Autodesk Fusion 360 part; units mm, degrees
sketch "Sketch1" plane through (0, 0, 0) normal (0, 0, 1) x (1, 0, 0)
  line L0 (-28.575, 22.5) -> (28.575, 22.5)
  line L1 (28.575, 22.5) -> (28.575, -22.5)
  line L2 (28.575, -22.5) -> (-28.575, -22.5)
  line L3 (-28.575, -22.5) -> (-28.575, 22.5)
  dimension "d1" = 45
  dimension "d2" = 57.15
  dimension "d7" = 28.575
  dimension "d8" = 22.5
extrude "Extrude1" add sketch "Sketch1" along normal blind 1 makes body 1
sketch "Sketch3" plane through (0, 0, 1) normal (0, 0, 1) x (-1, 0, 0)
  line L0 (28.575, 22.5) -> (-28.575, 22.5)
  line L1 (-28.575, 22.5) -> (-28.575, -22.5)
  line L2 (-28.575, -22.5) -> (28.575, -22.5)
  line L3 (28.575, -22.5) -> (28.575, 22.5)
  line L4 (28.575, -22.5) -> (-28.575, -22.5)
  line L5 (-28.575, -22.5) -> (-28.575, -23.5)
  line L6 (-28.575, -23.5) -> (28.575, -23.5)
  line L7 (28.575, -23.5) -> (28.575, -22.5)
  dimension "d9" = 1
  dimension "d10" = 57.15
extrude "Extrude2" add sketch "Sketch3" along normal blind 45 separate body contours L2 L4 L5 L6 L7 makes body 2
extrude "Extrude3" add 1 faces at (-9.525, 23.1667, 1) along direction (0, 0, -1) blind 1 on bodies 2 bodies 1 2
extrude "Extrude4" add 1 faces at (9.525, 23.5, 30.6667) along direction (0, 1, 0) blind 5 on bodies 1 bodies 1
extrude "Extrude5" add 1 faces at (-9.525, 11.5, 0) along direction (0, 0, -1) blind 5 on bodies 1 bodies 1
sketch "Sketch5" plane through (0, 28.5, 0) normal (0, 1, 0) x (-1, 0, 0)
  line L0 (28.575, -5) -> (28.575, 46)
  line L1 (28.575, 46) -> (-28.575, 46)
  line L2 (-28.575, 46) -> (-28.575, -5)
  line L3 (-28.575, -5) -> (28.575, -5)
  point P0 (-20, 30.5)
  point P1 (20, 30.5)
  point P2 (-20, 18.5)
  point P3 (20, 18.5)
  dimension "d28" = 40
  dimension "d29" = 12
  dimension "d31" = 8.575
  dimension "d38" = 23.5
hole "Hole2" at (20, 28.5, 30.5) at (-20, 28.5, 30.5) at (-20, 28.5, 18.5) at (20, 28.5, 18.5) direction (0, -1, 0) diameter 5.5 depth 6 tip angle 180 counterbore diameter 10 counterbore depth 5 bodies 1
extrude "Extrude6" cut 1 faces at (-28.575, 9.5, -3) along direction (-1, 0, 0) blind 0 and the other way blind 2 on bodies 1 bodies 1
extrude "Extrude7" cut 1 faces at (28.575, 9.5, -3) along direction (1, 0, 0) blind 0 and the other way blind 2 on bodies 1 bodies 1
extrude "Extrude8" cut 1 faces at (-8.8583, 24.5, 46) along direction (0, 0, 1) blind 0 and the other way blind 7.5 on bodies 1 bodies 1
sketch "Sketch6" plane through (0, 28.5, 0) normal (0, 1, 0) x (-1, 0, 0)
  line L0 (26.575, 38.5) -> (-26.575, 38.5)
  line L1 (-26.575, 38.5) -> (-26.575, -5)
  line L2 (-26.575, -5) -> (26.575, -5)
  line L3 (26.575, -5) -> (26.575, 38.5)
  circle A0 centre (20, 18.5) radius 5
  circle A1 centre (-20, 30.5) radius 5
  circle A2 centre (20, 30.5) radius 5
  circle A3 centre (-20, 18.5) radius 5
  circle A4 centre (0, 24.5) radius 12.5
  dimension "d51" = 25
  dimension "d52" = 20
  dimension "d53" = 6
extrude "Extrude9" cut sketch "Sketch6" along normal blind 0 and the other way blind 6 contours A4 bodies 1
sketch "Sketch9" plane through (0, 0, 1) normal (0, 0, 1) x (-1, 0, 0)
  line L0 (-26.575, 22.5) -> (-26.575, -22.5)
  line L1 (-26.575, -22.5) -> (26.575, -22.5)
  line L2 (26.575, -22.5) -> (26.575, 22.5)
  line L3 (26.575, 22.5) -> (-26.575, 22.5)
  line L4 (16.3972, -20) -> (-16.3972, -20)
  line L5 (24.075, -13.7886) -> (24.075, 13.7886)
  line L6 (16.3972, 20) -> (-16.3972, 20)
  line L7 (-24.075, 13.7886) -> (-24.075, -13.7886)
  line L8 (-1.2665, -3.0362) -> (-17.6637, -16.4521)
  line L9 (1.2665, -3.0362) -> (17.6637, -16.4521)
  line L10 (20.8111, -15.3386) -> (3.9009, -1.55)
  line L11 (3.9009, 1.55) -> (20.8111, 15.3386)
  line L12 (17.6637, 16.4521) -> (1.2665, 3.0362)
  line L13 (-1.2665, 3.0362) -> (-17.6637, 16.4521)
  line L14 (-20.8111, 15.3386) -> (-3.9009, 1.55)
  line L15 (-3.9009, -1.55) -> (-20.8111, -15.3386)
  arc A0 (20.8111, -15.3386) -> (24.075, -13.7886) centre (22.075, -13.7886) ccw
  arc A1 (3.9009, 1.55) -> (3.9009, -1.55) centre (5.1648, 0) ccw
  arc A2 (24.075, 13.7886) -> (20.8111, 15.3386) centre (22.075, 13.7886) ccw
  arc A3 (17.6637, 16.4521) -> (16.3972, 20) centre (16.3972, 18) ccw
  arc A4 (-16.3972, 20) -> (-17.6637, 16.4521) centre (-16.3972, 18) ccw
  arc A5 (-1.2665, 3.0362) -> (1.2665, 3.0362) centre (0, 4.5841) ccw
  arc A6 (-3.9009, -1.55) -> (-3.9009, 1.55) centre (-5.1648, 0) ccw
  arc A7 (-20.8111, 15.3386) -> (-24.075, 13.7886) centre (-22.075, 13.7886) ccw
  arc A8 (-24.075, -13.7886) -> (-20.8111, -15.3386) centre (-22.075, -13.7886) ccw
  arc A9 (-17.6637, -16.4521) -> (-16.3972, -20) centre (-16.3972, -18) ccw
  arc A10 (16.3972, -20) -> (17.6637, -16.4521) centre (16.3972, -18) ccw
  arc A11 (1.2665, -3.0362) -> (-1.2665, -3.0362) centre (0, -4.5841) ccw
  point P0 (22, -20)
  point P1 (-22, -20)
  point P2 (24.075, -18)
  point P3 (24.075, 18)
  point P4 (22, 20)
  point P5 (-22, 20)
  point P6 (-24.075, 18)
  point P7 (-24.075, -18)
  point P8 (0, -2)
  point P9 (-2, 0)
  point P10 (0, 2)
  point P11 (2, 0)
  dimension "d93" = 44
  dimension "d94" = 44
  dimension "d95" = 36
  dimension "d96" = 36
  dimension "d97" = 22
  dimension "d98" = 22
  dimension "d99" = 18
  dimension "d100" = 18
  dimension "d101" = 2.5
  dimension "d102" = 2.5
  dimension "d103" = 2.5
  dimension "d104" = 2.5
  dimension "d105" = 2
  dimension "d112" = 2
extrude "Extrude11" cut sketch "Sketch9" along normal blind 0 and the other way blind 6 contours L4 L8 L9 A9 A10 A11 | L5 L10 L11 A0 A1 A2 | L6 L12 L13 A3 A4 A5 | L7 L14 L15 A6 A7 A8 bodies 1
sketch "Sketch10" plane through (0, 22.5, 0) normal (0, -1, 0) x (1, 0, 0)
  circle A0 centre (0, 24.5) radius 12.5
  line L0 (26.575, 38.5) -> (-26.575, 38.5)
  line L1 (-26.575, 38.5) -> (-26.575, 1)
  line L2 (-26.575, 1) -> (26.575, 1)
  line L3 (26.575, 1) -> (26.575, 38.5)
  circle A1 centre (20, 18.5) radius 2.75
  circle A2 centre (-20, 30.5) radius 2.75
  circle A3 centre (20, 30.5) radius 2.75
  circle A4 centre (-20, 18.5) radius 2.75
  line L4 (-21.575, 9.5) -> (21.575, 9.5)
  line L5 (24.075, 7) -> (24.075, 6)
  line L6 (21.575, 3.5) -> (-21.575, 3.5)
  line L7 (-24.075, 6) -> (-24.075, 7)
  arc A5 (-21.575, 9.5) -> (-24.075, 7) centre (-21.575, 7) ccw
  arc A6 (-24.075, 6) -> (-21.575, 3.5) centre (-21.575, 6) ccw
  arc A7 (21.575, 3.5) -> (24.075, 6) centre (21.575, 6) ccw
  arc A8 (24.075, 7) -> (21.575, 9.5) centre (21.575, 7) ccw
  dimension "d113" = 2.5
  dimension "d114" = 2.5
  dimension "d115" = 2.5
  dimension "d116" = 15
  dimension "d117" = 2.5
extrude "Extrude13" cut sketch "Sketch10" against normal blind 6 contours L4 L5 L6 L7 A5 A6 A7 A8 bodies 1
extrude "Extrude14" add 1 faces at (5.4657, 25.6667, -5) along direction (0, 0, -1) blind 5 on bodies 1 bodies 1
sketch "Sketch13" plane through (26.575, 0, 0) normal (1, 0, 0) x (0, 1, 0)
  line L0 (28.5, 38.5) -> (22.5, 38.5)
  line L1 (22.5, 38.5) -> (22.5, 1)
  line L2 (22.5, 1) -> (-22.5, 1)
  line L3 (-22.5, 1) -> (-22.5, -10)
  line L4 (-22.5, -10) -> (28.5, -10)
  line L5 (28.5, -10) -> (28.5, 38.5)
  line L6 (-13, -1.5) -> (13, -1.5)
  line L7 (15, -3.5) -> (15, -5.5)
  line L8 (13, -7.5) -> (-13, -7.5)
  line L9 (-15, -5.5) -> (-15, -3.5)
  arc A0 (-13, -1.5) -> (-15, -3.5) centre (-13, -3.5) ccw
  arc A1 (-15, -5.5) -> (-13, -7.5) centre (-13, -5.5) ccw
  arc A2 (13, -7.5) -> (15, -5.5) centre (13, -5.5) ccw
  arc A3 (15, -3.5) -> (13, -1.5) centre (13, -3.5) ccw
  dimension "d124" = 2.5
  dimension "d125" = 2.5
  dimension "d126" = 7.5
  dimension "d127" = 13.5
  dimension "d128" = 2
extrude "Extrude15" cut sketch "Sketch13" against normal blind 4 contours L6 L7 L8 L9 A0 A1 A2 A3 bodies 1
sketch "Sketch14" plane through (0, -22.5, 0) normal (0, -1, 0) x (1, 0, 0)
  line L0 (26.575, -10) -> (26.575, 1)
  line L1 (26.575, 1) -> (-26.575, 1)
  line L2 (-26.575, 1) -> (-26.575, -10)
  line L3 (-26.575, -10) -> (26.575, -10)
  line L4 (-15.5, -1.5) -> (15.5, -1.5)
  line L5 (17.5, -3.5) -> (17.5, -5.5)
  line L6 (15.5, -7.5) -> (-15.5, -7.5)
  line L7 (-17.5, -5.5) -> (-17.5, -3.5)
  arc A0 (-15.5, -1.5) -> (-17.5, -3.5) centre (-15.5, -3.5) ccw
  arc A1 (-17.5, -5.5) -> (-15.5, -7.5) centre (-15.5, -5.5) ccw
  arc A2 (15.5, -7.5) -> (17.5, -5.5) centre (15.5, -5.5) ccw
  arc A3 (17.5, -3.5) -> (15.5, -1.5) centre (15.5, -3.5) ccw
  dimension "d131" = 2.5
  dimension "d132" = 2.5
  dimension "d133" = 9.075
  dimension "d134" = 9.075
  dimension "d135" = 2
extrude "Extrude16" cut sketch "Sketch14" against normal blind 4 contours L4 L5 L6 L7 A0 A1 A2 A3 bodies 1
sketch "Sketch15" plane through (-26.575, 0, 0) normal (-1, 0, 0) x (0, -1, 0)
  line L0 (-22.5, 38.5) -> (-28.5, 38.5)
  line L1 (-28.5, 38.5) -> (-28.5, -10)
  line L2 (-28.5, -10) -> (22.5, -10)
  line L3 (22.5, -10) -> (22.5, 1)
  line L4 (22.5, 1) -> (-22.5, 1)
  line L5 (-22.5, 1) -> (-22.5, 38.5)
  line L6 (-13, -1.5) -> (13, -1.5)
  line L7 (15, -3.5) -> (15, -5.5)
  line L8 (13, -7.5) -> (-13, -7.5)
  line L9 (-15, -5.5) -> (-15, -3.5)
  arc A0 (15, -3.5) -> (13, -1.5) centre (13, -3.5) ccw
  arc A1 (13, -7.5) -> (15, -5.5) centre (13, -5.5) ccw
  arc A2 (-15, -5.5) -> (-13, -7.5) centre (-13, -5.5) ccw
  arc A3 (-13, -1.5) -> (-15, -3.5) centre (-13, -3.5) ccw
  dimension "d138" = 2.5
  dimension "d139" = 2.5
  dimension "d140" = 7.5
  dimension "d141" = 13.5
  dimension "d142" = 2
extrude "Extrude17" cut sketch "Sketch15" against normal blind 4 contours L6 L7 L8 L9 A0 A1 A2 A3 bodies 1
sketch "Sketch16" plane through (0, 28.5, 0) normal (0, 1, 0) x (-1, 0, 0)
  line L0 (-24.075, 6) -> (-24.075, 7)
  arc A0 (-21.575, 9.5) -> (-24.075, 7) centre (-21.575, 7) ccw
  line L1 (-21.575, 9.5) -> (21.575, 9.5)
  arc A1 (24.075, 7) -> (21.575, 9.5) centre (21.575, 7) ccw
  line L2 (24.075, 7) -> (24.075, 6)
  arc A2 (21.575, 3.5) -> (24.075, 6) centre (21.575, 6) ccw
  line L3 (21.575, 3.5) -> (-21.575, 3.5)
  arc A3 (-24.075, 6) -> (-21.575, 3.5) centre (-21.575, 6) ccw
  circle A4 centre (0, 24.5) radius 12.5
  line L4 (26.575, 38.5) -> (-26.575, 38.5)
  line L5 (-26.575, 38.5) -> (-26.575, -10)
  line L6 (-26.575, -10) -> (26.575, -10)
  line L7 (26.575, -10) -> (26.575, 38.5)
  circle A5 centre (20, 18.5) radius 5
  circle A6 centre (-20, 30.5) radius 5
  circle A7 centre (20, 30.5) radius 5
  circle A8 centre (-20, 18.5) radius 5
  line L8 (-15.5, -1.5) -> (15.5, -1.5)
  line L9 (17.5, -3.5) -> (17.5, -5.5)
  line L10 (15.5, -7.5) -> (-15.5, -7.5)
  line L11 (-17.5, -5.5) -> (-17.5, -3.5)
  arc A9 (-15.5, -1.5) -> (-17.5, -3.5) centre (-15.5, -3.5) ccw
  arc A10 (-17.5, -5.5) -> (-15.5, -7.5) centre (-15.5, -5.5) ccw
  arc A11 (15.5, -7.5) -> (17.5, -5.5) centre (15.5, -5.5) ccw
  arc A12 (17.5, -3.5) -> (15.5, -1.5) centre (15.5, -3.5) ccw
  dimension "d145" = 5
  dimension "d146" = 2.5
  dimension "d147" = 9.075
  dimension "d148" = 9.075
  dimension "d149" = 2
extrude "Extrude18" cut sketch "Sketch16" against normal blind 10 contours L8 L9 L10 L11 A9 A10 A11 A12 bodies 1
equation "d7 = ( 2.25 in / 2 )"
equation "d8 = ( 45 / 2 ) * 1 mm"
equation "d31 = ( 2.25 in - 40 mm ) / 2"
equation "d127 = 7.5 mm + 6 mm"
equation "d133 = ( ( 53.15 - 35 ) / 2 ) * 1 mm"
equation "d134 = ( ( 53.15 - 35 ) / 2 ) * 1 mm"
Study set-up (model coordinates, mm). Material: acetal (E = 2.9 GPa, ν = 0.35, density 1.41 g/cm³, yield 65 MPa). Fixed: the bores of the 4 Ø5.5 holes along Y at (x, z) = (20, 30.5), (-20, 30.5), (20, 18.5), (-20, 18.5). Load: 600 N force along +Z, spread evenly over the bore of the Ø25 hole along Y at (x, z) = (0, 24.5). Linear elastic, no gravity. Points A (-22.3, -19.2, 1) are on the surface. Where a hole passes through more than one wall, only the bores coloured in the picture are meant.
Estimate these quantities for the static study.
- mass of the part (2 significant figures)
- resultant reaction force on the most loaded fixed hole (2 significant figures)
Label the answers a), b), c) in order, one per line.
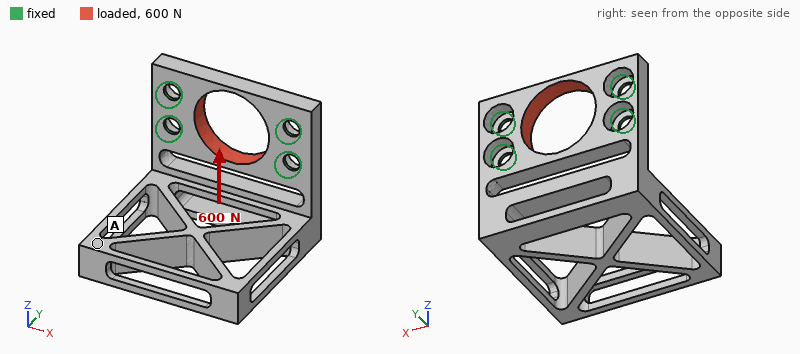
a) 22 g
b) 170 N
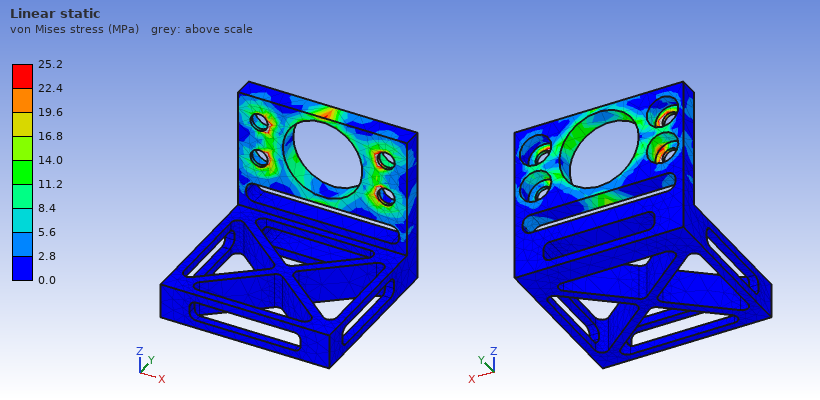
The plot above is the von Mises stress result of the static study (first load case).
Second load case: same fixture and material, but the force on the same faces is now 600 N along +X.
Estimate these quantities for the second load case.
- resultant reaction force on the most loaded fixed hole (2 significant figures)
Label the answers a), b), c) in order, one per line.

a) 150 N
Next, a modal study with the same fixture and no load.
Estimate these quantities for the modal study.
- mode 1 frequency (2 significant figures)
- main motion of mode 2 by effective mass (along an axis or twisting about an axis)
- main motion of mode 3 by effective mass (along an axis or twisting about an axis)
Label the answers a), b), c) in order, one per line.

a) 190 Hz
b) along X
c) along Y
